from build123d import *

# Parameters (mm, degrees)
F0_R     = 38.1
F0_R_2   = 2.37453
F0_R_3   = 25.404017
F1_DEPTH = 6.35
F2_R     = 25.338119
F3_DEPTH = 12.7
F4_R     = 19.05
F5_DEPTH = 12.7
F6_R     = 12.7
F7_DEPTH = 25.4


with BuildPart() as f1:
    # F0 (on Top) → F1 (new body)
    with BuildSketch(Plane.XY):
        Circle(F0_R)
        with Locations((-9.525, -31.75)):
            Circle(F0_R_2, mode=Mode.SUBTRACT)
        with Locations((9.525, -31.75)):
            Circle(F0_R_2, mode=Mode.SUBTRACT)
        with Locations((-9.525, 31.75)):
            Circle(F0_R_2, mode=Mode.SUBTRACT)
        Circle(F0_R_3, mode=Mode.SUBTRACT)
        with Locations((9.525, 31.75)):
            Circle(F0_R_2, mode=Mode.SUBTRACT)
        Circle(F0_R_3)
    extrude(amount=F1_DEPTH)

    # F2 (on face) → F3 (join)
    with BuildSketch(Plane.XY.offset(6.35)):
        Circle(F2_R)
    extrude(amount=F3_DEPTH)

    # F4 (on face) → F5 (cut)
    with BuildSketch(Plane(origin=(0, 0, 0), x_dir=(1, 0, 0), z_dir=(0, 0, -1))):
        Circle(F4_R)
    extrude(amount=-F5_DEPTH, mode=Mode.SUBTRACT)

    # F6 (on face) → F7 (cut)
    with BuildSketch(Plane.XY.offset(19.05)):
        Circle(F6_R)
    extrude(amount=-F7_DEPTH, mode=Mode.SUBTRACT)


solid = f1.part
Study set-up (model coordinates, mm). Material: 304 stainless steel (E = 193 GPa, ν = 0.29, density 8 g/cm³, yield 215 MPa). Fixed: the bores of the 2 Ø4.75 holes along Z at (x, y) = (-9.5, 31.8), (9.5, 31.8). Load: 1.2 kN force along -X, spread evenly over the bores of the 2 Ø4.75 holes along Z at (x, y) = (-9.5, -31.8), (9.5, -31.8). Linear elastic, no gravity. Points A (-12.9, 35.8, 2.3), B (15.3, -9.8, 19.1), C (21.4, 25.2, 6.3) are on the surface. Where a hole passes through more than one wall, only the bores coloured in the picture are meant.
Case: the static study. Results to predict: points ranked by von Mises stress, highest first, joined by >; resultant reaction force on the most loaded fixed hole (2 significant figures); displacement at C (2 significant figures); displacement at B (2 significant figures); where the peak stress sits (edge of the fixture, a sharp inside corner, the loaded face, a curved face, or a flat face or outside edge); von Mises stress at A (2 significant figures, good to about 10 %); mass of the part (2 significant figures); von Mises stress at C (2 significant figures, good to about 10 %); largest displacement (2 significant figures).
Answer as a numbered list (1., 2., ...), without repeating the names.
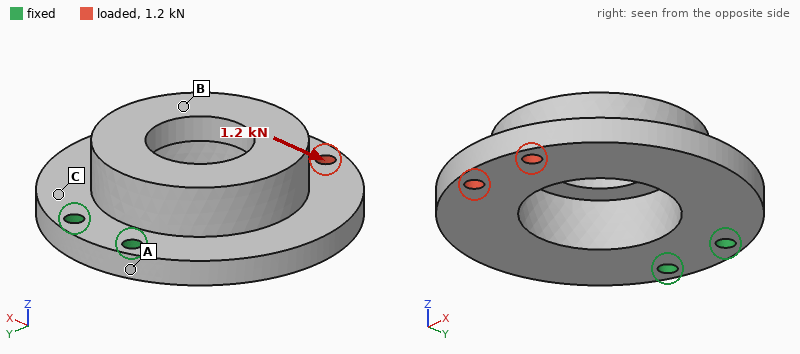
1. A > C > B
2. 3.1 kN
3. 8.3 µm
4. 23 µm
5. edge of the fixture
6. 62 MPa
7. 290 g
8. 33 MPa
9. 45 µm
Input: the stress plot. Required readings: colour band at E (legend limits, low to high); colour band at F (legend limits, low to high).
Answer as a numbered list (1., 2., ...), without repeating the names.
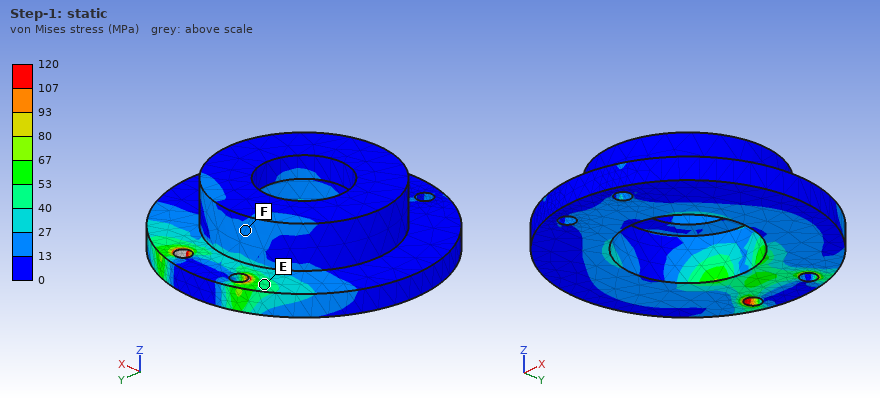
1. 40 to 53 MPa
2. 13 to 27 MPa
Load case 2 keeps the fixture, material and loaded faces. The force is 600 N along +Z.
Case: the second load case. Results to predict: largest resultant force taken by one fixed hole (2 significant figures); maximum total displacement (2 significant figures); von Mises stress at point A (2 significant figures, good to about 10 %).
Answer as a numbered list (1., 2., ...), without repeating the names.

1. 690 N
2. 0.19 mm
3. 67 MPa
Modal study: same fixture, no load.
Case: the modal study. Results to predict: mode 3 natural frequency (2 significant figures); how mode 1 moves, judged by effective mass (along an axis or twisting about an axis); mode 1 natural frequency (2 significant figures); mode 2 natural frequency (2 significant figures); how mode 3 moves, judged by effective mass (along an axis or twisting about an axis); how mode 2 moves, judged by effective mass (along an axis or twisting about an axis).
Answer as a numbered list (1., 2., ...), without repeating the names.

1. 3300 Hz
2. along Z
3. 1000 Hz
4. 2500 Hz
5. along X
6. along X
